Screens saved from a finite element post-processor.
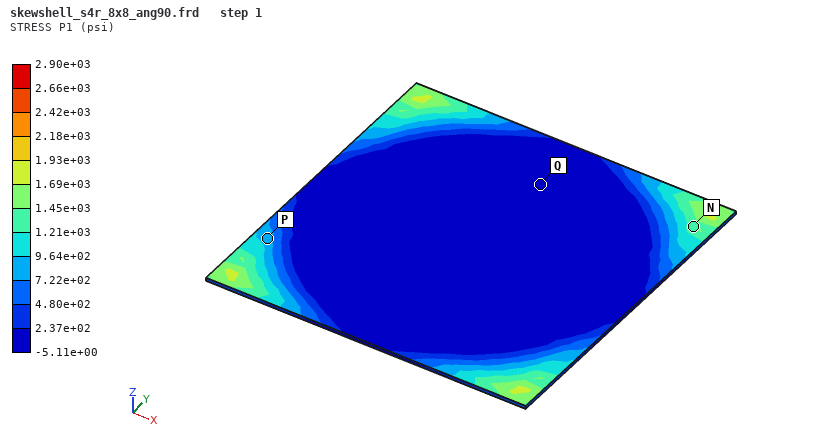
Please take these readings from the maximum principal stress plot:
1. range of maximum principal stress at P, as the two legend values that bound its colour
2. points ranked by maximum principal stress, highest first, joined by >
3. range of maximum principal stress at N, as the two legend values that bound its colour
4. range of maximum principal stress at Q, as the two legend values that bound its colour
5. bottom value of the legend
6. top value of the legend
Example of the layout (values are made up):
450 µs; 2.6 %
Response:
7.22e+02 to 9.64e+02 psi; N > P > Q; 1.21e+03 to 1.45e+03 psi; -5.11e+00 to 2.37e+02 psi; -5.11e+00 psi; 2.90e+03 psi
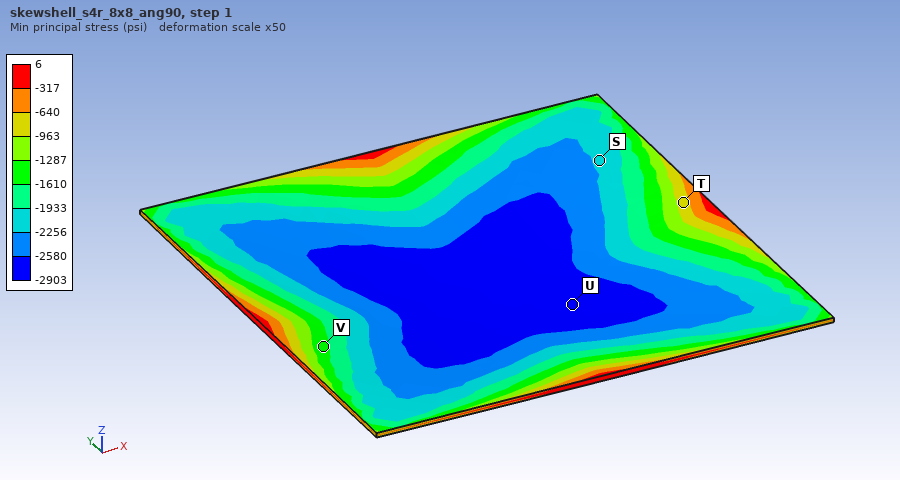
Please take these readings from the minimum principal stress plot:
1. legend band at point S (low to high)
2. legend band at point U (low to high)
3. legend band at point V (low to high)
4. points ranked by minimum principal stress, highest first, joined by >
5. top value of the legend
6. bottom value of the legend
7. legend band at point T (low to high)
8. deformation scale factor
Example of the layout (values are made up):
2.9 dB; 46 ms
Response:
-2256 to -1933 psi; -2903 to -2580 psi; -1610 to -1287 psi; T > V > S > U; 6 psi; -2903 psi; -963 to -640 psi; 50
